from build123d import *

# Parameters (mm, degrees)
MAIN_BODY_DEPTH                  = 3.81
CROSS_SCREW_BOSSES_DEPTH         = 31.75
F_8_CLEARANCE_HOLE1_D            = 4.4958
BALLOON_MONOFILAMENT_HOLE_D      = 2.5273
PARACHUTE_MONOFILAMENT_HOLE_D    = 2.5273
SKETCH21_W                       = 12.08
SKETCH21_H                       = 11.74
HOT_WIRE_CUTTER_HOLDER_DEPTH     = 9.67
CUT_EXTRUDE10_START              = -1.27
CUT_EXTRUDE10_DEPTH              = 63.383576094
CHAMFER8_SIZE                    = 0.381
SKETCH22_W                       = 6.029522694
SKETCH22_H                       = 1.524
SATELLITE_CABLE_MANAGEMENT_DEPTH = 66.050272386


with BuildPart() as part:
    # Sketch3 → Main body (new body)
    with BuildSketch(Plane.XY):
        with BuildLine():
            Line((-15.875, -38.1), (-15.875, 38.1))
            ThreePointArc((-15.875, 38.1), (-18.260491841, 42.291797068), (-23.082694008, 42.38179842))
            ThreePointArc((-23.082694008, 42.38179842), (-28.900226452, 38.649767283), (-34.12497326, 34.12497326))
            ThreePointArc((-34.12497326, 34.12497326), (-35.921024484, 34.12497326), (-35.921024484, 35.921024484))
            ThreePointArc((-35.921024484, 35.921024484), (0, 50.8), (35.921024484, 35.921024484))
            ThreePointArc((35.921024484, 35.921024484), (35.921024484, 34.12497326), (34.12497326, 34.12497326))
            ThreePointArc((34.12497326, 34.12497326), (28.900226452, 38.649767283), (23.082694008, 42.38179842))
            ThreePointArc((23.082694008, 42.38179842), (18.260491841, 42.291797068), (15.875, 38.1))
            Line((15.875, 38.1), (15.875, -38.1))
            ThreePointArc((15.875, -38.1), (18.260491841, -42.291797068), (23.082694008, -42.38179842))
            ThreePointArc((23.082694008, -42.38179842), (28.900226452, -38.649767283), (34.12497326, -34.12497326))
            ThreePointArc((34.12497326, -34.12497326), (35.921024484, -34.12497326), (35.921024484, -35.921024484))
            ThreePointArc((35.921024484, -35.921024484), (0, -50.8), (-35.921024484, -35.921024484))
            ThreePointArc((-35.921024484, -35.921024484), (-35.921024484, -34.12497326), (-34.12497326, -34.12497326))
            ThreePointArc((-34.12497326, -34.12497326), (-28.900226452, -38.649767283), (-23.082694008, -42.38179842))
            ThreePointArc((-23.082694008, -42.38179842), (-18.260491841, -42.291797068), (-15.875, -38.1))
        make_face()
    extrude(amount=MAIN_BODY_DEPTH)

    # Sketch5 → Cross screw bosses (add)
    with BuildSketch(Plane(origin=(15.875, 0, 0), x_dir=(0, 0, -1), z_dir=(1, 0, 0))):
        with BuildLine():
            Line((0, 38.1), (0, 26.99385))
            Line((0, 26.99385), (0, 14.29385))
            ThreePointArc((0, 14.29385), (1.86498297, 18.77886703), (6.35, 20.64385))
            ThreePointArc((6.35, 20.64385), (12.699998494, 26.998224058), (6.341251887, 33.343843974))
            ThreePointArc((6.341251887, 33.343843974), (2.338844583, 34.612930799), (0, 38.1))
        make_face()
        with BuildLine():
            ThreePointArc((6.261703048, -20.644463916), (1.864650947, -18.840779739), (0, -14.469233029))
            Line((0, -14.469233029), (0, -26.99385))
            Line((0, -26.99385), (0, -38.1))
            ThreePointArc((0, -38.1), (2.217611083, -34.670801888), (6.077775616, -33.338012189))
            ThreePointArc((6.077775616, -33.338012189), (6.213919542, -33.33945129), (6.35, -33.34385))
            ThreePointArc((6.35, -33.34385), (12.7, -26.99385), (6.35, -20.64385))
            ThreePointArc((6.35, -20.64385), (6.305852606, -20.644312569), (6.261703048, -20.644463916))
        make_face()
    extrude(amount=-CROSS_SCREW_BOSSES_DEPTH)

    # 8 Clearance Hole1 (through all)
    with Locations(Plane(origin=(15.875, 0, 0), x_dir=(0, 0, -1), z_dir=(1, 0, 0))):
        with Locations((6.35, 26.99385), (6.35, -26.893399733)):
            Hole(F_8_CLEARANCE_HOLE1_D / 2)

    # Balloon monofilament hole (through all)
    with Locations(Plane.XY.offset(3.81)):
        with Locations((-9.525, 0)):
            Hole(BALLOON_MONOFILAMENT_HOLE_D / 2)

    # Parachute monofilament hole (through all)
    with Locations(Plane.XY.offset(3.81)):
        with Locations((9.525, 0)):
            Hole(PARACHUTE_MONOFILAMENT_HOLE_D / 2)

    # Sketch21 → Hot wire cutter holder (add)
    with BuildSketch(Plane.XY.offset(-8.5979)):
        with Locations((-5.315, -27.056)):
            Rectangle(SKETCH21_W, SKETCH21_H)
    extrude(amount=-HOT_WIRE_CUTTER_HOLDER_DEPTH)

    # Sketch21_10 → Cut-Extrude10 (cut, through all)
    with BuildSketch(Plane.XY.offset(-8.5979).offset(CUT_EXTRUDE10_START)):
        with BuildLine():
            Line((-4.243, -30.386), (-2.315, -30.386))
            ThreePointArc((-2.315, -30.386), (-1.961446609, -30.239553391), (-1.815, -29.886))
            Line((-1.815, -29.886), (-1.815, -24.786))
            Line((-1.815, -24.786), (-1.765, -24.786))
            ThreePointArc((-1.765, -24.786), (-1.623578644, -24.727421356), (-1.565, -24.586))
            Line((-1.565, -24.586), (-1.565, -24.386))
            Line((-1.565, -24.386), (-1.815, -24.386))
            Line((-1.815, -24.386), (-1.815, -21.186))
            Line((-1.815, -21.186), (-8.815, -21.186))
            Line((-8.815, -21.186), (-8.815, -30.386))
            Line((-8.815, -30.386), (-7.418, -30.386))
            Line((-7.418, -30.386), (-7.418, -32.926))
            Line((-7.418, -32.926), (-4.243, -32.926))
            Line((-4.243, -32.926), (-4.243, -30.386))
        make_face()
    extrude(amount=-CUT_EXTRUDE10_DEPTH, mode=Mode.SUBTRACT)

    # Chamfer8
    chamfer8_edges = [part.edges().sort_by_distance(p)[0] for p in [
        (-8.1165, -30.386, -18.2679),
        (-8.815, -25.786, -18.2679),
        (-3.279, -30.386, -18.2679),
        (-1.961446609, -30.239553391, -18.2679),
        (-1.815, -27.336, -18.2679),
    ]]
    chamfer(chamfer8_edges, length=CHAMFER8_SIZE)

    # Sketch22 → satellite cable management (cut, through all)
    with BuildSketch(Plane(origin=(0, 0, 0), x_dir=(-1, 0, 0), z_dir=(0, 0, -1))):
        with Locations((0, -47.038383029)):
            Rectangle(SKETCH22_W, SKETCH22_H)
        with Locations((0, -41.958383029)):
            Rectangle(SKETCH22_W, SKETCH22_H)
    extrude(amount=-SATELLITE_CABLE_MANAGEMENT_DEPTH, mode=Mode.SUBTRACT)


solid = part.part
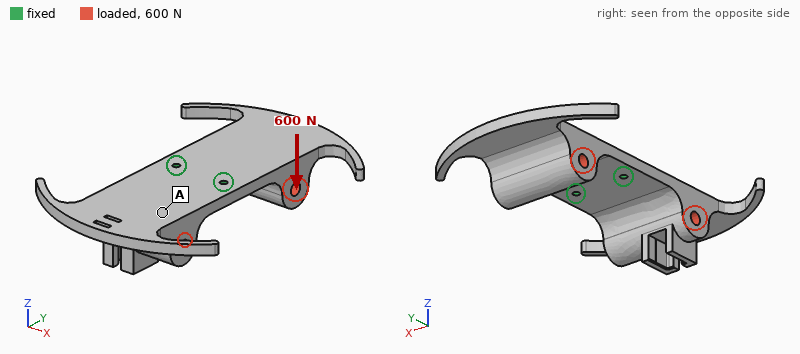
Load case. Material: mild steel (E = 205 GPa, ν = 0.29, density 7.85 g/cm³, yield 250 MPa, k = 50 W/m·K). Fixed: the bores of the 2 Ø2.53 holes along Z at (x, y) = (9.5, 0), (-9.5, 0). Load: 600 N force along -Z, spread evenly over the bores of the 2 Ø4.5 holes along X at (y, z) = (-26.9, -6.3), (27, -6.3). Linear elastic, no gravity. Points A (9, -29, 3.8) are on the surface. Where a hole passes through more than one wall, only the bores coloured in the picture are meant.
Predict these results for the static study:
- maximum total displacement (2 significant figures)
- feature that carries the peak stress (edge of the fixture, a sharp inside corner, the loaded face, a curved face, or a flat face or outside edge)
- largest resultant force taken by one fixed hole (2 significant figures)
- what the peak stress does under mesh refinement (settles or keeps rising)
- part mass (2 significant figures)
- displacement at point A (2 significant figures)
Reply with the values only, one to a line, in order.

0.13 mm
edge of the fixture
300 N
keeps rising
180 g
0.065 mm
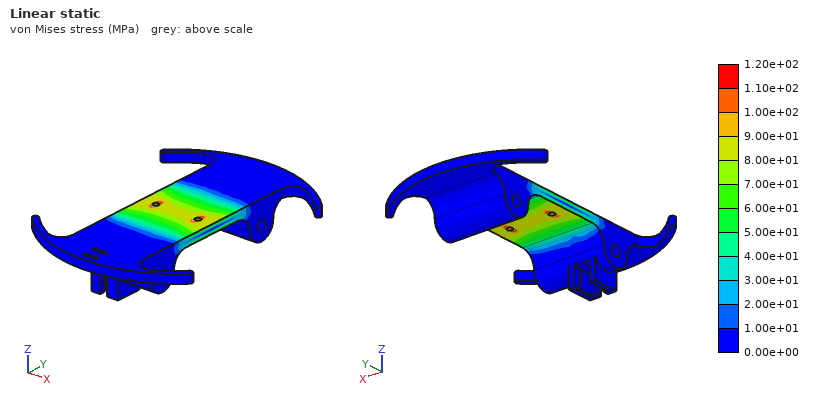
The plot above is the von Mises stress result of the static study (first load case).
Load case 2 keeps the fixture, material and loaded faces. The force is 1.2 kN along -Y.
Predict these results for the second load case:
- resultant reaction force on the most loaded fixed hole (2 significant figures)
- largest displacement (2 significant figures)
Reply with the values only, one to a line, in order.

600 N
0.14 mm
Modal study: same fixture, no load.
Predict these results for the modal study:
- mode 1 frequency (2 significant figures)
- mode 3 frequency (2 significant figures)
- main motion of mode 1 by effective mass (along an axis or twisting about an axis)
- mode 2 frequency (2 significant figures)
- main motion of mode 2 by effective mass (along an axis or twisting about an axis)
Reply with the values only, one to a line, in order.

890 Hz
3100 Hz
twisting about X
1000 Hz
along Z
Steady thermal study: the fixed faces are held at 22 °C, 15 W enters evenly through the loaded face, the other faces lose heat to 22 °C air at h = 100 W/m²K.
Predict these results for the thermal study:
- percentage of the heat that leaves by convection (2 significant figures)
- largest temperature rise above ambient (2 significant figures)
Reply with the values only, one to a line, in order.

66 %
15 K
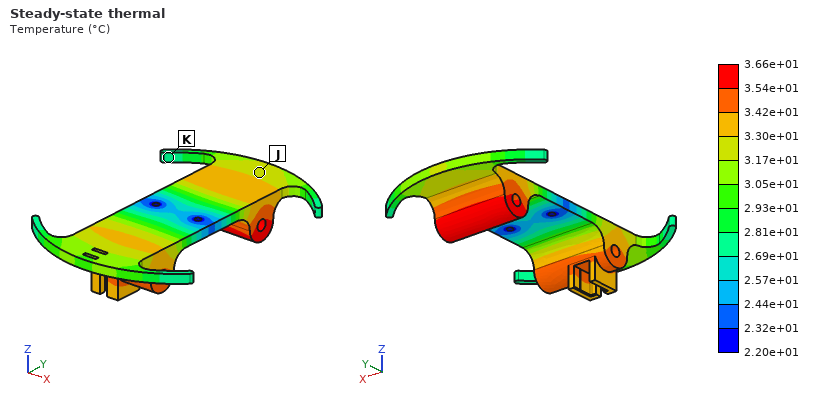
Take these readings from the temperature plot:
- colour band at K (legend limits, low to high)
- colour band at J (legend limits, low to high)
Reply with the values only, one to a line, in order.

2.69e+01 to 2.81e+01 °C
3.17e+01 to 3.30e+01 °C
